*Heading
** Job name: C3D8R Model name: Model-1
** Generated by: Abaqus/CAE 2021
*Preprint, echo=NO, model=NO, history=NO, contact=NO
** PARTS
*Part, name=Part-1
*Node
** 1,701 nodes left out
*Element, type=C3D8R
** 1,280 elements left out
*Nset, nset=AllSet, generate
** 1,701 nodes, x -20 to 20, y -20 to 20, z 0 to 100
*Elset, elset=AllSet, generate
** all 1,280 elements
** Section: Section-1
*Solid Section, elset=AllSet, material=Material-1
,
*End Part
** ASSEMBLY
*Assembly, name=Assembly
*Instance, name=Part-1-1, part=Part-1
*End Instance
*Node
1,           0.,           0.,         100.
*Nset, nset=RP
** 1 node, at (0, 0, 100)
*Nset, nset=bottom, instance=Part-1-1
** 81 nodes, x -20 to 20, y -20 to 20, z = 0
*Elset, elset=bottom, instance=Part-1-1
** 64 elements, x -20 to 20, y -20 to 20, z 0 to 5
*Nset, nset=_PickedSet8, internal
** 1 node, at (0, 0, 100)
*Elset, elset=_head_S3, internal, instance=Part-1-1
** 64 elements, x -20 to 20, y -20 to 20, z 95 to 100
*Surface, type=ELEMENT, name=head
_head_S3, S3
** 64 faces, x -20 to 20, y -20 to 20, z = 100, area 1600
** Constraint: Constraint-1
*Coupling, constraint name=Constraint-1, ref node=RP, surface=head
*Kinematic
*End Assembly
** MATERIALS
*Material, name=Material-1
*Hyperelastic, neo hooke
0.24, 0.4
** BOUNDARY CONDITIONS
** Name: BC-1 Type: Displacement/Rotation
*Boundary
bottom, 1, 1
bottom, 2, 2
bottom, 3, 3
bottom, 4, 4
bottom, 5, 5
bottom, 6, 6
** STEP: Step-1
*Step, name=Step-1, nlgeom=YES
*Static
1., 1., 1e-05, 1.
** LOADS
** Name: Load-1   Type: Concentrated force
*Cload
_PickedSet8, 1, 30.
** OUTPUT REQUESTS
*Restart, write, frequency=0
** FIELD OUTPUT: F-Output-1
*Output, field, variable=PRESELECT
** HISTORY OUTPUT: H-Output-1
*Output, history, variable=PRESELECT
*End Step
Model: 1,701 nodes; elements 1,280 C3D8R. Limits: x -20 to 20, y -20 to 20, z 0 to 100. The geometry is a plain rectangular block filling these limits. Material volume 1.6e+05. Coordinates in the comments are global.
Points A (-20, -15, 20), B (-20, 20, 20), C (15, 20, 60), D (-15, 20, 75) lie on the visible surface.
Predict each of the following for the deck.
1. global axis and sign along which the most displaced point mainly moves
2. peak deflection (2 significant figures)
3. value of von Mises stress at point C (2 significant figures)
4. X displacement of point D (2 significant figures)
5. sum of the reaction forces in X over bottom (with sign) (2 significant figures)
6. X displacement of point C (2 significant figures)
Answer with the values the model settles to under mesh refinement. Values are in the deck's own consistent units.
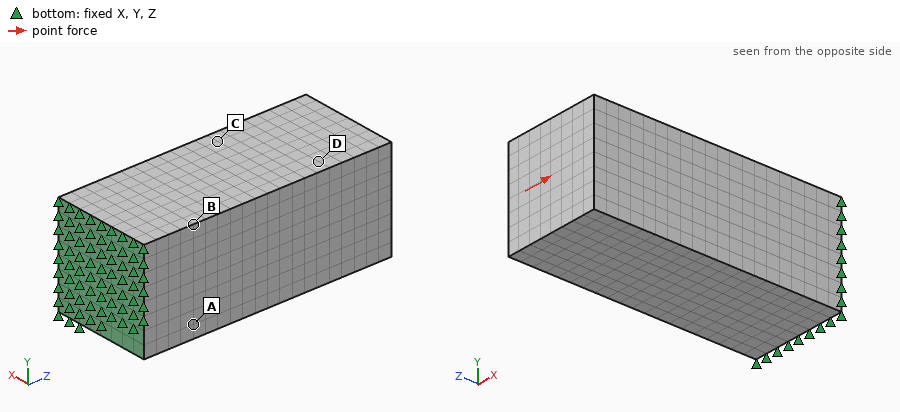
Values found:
+X
35
0.072
23
-30
14
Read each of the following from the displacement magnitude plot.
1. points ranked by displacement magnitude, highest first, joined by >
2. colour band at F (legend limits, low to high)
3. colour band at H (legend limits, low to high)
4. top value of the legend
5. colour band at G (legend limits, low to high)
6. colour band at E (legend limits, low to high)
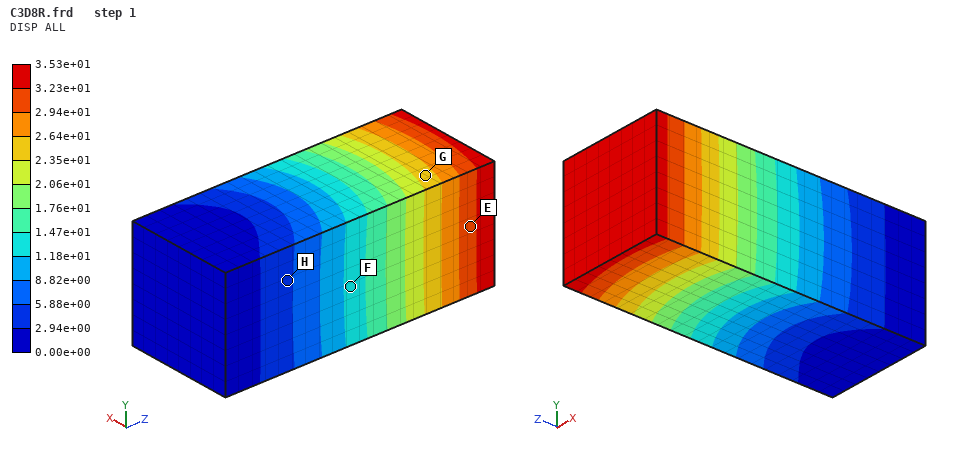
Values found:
E > G > F > H
1.18e+01 to 1.47e+01
2.94e+00 to 5.88e+00
3.53e+01
2.35e+01 to 2.64e+01
2.94e+01 to 3.23e+01
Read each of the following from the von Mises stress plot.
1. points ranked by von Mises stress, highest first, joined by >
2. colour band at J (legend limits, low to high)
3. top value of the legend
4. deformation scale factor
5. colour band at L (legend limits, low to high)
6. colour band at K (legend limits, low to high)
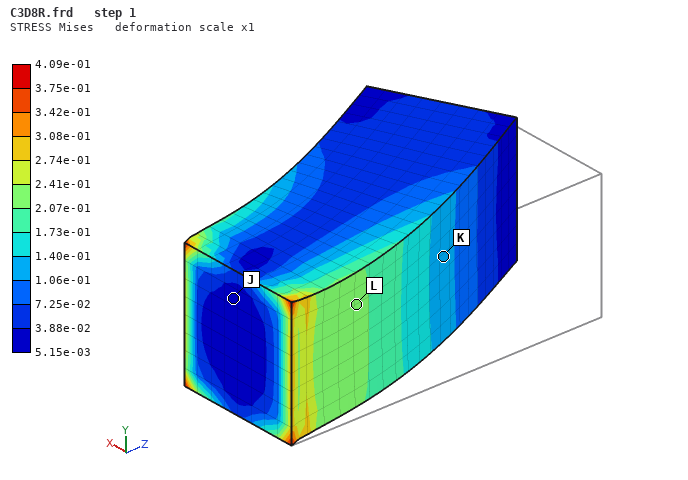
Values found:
L > K > J
5.15e-03 to 3.88e-02
4.09e-01
1
2.07e-01 to 2.41e-01
1.06e-01 to 1.40e-01
